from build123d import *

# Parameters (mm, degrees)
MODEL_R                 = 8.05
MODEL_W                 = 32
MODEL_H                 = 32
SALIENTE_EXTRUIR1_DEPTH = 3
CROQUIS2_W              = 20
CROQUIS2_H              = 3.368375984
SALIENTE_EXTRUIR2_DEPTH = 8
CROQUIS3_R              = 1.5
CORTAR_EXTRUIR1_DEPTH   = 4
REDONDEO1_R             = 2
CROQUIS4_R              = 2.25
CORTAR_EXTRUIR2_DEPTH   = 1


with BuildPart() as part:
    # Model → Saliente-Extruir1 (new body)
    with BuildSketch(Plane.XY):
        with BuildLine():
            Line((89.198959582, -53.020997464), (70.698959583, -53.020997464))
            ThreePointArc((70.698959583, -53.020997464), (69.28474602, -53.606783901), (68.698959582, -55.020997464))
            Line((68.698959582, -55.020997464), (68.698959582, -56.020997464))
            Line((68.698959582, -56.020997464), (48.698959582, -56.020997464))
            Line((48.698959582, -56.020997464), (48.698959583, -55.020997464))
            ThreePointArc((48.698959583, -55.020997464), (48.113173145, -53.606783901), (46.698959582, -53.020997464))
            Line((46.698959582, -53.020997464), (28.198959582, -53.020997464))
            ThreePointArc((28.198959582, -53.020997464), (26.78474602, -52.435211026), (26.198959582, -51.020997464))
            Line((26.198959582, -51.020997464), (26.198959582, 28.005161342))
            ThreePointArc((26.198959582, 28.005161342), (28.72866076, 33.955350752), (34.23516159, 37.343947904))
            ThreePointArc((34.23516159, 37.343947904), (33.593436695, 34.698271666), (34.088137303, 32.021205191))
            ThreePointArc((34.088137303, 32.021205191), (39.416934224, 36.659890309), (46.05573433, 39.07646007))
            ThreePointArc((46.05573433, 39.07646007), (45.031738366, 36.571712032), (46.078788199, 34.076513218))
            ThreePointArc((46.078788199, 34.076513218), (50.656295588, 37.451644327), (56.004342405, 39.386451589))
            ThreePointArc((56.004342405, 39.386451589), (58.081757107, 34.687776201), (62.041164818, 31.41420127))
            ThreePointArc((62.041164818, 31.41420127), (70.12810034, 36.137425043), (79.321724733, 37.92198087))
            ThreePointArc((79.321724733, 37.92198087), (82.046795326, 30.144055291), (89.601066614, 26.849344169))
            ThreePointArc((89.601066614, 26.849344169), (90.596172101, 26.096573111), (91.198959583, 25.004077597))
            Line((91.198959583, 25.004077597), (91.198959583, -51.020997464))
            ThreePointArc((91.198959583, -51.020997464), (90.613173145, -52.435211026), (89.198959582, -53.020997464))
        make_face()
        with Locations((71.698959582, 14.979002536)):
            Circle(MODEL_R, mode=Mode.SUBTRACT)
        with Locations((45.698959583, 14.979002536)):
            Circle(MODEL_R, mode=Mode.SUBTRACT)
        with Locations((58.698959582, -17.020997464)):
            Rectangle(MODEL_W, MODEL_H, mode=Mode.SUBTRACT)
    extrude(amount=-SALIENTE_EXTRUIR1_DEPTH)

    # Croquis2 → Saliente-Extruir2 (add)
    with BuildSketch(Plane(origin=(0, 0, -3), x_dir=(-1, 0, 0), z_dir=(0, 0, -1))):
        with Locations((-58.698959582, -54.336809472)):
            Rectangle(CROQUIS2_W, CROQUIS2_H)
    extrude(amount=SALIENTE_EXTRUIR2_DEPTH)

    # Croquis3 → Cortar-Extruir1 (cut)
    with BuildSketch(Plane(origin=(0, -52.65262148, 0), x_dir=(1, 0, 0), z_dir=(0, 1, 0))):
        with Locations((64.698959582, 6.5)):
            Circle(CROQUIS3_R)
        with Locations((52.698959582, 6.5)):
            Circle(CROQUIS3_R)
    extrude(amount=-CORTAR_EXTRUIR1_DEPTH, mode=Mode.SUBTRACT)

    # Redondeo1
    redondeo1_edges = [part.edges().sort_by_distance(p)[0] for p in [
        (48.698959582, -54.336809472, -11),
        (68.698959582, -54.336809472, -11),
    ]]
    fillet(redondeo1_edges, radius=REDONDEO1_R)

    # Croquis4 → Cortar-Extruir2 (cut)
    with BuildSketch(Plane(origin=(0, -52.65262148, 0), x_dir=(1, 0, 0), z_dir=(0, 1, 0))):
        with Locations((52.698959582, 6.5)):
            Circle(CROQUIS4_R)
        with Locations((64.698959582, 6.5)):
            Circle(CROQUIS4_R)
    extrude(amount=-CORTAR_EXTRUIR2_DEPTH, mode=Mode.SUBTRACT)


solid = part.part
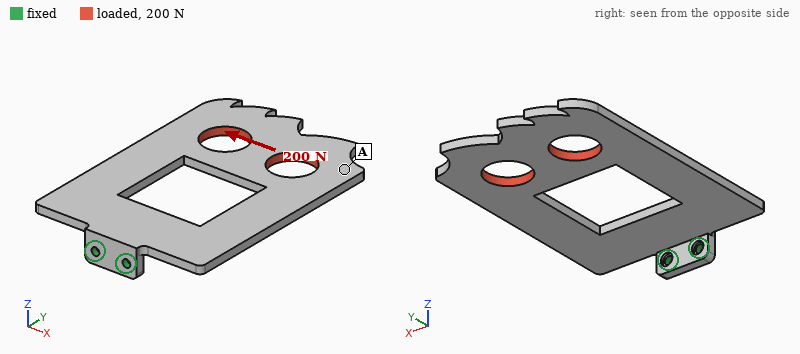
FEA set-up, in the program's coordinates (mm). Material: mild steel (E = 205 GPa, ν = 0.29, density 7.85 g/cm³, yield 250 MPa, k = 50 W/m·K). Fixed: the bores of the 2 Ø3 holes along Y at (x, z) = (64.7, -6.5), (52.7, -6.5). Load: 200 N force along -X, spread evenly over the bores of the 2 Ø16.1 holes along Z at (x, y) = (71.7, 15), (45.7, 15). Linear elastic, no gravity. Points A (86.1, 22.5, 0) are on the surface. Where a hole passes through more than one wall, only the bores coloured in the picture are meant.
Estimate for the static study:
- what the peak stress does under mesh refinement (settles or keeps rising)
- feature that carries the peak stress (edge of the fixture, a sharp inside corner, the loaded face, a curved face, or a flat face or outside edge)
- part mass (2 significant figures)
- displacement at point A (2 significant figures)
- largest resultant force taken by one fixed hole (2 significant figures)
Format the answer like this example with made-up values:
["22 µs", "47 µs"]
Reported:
["keeps rising", "edge of the fixture", "110 g", "0.12 mm", "1.0 kN"]
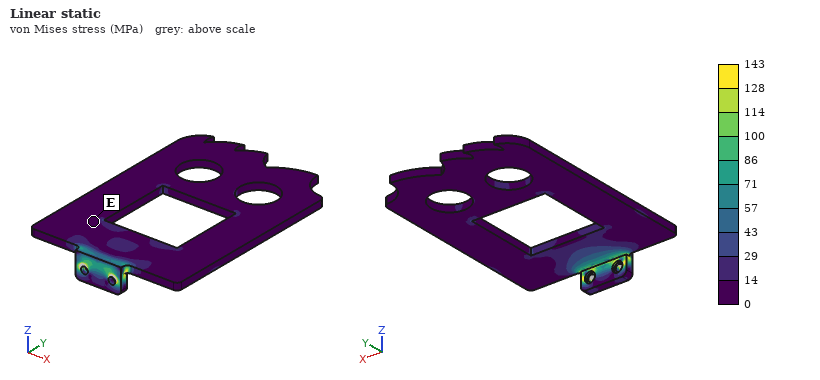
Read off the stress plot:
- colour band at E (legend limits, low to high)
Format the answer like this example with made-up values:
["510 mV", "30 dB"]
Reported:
["0 to 14 MPa"]
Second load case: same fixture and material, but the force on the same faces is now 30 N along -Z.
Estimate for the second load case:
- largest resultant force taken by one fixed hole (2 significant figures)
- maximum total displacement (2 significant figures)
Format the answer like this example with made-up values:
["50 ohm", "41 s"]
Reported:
["36 N", "0.43 mm"]
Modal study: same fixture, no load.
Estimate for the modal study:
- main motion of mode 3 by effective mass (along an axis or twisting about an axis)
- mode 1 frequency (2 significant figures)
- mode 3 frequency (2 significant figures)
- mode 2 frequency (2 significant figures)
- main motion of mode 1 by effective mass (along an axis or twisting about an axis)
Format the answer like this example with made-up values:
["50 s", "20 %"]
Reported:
["along X", "210 Hz", "920 Hz", "630 Hz", "along Z"]
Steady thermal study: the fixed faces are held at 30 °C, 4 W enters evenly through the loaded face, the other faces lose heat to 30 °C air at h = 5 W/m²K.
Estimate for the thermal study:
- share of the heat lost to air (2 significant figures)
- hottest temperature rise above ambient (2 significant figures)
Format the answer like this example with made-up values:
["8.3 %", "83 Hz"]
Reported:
["37 %", "48 K"]
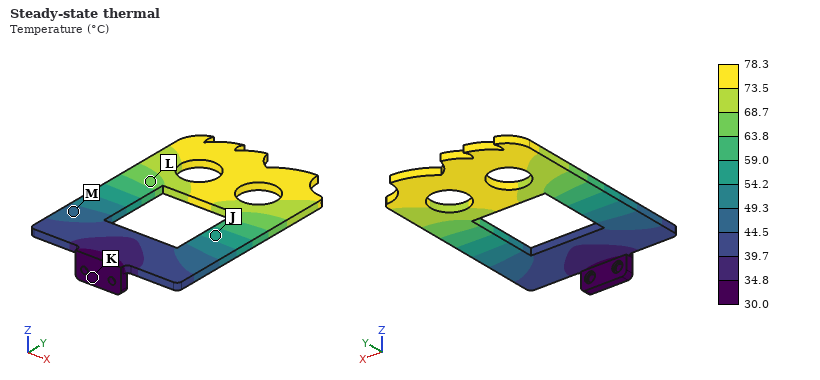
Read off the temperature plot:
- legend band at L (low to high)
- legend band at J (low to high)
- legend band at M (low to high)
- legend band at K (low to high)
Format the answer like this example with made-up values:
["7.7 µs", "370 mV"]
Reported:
["63.8 to 68.7 °C", "54.2 to 59.0 °C", "44.5 to 49.3 °C", "30.0 to 34.8 °C"]
